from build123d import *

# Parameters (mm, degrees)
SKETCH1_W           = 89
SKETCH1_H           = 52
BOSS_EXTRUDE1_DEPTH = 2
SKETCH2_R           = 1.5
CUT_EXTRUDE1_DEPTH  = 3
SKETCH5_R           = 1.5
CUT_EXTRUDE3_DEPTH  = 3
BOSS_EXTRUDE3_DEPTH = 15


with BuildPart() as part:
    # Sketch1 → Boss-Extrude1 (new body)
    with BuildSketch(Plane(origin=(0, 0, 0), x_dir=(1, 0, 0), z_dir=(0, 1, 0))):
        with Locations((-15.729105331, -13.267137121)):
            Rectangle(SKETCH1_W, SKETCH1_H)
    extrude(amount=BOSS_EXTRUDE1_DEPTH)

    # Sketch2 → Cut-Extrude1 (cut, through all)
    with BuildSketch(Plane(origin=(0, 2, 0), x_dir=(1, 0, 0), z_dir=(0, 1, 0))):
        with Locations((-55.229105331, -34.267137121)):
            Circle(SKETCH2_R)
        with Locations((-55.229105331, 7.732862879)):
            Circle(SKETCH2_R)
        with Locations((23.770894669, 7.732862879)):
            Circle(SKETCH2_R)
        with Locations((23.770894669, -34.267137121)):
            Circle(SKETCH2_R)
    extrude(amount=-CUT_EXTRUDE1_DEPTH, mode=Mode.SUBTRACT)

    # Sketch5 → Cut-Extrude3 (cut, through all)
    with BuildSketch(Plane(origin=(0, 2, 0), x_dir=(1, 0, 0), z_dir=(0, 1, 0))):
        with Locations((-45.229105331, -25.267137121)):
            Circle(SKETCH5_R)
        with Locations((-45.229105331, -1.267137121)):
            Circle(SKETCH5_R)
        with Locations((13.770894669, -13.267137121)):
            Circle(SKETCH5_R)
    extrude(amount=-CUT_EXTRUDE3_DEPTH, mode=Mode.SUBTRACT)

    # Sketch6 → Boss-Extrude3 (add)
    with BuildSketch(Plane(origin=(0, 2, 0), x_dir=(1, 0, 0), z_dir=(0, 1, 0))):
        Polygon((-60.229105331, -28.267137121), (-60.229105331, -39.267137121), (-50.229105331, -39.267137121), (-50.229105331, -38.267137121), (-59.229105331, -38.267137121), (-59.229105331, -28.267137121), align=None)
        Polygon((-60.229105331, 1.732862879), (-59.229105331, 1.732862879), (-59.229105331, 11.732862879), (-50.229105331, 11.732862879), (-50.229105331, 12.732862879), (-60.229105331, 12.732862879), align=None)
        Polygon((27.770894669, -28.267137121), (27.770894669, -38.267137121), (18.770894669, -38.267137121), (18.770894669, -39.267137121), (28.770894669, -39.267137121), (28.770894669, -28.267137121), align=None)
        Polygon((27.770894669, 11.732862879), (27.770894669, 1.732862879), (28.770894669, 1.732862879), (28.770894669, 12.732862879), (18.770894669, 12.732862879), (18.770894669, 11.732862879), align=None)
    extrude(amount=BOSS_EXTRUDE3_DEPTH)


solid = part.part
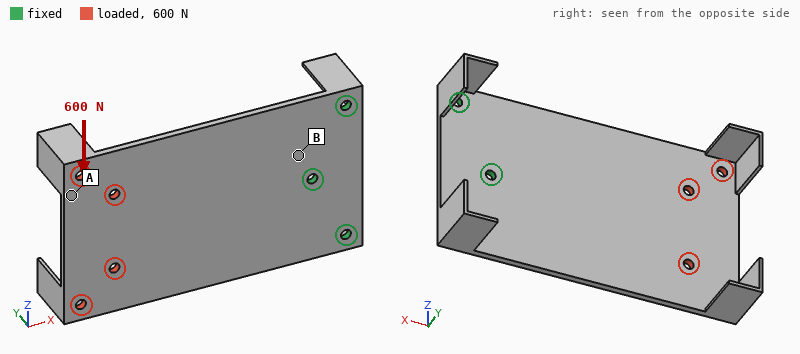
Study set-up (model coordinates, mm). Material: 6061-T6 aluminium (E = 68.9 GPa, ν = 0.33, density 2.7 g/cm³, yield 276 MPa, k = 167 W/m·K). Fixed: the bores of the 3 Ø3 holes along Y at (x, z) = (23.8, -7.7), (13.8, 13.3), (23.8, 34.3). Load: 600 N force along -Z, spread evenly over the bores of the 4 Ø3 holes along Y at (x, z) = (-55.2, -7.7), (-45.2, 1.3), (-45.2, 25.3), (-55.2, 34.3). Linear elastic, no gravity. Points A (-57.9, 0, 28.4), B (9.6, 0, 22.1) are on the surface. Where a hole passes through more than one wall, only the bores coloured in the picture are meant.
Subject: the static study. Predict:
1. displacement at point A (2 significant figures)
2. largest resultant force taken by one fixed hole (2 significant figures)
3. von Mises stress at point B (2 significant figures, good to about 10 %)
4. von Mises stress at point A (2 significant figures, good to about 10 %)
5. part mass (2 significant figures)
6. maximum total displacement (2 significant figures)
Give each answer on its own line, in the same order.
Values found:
81 µm
910 N
16 MPa
6.6 MPa
28 g
88 µm
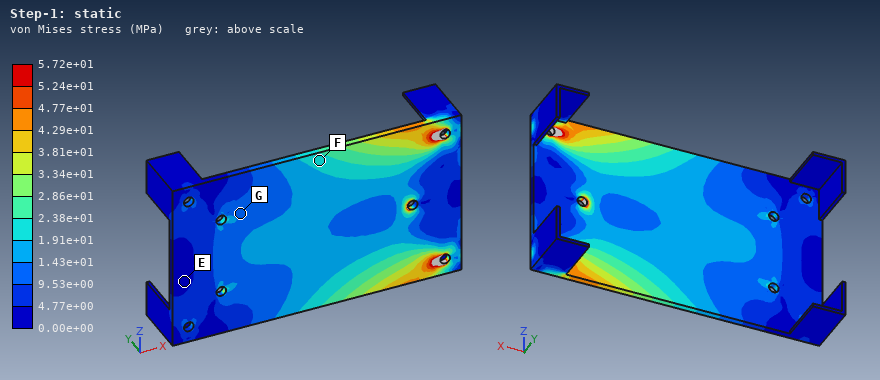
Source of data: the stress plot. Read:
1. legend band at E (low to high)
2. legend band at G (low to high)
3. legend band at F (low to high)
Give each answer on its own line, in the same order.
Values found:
0.00e+00 to 4.77e+00 MPa
9.53e+00 to 1.43e+01 MPa
1.91e+01 to 2.38e+01 MPa
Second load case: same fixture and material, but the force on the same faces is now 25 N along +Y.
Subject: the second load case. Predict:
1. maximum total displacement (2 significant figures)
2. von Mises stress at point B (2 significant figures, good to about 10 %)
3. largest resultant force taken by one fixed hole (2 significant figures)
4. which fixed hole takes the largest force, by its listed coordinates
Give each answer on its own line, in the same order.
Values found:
1.2 mm
39 MPa
72 N
(13.8, 13.3)
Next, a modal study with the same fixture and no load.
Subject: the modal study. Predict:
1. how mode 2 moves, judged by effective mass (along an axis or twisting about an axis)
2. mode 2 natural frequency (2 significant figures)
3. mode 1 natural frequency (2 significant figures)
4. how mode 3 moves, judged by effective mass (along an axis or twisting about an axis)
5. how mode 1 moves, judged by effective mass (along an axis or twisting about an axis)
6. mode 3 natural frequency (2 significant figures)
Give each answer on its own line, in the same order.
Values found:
twisting about X
710 Hz
260 Hz
along Y
along Y
1500 Hz
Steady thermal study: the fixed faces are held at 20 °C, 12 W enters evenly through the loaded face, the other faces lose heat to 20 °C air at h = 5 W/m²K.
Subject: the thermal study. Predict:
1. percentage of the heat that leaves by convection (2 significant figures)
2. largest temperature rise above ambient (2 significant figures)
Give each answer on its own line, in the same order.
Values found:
12 %
48 K
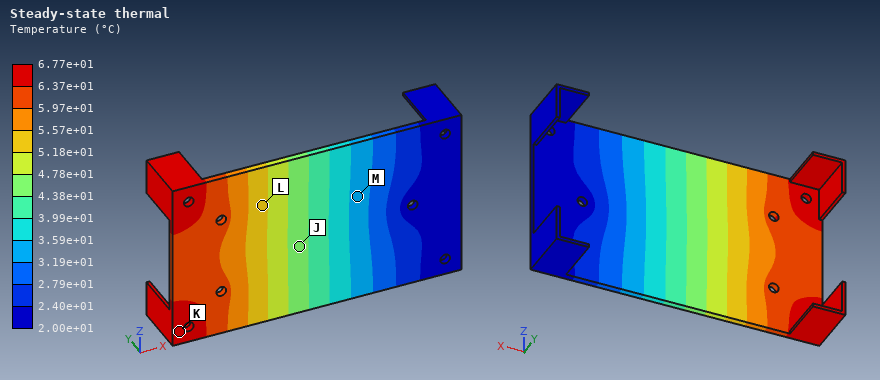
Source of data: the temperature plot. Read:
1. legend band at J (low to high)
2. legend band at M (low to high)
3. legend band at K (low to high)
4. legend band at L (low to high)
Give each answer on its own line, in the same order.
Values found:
4.38e+01 to 4.78e+01 °C
3.19e+01 to 3.59e+01 °C
6.37e+01 to 6.77e+01 °C
5.18e+01 to 5.57e+01 °C
